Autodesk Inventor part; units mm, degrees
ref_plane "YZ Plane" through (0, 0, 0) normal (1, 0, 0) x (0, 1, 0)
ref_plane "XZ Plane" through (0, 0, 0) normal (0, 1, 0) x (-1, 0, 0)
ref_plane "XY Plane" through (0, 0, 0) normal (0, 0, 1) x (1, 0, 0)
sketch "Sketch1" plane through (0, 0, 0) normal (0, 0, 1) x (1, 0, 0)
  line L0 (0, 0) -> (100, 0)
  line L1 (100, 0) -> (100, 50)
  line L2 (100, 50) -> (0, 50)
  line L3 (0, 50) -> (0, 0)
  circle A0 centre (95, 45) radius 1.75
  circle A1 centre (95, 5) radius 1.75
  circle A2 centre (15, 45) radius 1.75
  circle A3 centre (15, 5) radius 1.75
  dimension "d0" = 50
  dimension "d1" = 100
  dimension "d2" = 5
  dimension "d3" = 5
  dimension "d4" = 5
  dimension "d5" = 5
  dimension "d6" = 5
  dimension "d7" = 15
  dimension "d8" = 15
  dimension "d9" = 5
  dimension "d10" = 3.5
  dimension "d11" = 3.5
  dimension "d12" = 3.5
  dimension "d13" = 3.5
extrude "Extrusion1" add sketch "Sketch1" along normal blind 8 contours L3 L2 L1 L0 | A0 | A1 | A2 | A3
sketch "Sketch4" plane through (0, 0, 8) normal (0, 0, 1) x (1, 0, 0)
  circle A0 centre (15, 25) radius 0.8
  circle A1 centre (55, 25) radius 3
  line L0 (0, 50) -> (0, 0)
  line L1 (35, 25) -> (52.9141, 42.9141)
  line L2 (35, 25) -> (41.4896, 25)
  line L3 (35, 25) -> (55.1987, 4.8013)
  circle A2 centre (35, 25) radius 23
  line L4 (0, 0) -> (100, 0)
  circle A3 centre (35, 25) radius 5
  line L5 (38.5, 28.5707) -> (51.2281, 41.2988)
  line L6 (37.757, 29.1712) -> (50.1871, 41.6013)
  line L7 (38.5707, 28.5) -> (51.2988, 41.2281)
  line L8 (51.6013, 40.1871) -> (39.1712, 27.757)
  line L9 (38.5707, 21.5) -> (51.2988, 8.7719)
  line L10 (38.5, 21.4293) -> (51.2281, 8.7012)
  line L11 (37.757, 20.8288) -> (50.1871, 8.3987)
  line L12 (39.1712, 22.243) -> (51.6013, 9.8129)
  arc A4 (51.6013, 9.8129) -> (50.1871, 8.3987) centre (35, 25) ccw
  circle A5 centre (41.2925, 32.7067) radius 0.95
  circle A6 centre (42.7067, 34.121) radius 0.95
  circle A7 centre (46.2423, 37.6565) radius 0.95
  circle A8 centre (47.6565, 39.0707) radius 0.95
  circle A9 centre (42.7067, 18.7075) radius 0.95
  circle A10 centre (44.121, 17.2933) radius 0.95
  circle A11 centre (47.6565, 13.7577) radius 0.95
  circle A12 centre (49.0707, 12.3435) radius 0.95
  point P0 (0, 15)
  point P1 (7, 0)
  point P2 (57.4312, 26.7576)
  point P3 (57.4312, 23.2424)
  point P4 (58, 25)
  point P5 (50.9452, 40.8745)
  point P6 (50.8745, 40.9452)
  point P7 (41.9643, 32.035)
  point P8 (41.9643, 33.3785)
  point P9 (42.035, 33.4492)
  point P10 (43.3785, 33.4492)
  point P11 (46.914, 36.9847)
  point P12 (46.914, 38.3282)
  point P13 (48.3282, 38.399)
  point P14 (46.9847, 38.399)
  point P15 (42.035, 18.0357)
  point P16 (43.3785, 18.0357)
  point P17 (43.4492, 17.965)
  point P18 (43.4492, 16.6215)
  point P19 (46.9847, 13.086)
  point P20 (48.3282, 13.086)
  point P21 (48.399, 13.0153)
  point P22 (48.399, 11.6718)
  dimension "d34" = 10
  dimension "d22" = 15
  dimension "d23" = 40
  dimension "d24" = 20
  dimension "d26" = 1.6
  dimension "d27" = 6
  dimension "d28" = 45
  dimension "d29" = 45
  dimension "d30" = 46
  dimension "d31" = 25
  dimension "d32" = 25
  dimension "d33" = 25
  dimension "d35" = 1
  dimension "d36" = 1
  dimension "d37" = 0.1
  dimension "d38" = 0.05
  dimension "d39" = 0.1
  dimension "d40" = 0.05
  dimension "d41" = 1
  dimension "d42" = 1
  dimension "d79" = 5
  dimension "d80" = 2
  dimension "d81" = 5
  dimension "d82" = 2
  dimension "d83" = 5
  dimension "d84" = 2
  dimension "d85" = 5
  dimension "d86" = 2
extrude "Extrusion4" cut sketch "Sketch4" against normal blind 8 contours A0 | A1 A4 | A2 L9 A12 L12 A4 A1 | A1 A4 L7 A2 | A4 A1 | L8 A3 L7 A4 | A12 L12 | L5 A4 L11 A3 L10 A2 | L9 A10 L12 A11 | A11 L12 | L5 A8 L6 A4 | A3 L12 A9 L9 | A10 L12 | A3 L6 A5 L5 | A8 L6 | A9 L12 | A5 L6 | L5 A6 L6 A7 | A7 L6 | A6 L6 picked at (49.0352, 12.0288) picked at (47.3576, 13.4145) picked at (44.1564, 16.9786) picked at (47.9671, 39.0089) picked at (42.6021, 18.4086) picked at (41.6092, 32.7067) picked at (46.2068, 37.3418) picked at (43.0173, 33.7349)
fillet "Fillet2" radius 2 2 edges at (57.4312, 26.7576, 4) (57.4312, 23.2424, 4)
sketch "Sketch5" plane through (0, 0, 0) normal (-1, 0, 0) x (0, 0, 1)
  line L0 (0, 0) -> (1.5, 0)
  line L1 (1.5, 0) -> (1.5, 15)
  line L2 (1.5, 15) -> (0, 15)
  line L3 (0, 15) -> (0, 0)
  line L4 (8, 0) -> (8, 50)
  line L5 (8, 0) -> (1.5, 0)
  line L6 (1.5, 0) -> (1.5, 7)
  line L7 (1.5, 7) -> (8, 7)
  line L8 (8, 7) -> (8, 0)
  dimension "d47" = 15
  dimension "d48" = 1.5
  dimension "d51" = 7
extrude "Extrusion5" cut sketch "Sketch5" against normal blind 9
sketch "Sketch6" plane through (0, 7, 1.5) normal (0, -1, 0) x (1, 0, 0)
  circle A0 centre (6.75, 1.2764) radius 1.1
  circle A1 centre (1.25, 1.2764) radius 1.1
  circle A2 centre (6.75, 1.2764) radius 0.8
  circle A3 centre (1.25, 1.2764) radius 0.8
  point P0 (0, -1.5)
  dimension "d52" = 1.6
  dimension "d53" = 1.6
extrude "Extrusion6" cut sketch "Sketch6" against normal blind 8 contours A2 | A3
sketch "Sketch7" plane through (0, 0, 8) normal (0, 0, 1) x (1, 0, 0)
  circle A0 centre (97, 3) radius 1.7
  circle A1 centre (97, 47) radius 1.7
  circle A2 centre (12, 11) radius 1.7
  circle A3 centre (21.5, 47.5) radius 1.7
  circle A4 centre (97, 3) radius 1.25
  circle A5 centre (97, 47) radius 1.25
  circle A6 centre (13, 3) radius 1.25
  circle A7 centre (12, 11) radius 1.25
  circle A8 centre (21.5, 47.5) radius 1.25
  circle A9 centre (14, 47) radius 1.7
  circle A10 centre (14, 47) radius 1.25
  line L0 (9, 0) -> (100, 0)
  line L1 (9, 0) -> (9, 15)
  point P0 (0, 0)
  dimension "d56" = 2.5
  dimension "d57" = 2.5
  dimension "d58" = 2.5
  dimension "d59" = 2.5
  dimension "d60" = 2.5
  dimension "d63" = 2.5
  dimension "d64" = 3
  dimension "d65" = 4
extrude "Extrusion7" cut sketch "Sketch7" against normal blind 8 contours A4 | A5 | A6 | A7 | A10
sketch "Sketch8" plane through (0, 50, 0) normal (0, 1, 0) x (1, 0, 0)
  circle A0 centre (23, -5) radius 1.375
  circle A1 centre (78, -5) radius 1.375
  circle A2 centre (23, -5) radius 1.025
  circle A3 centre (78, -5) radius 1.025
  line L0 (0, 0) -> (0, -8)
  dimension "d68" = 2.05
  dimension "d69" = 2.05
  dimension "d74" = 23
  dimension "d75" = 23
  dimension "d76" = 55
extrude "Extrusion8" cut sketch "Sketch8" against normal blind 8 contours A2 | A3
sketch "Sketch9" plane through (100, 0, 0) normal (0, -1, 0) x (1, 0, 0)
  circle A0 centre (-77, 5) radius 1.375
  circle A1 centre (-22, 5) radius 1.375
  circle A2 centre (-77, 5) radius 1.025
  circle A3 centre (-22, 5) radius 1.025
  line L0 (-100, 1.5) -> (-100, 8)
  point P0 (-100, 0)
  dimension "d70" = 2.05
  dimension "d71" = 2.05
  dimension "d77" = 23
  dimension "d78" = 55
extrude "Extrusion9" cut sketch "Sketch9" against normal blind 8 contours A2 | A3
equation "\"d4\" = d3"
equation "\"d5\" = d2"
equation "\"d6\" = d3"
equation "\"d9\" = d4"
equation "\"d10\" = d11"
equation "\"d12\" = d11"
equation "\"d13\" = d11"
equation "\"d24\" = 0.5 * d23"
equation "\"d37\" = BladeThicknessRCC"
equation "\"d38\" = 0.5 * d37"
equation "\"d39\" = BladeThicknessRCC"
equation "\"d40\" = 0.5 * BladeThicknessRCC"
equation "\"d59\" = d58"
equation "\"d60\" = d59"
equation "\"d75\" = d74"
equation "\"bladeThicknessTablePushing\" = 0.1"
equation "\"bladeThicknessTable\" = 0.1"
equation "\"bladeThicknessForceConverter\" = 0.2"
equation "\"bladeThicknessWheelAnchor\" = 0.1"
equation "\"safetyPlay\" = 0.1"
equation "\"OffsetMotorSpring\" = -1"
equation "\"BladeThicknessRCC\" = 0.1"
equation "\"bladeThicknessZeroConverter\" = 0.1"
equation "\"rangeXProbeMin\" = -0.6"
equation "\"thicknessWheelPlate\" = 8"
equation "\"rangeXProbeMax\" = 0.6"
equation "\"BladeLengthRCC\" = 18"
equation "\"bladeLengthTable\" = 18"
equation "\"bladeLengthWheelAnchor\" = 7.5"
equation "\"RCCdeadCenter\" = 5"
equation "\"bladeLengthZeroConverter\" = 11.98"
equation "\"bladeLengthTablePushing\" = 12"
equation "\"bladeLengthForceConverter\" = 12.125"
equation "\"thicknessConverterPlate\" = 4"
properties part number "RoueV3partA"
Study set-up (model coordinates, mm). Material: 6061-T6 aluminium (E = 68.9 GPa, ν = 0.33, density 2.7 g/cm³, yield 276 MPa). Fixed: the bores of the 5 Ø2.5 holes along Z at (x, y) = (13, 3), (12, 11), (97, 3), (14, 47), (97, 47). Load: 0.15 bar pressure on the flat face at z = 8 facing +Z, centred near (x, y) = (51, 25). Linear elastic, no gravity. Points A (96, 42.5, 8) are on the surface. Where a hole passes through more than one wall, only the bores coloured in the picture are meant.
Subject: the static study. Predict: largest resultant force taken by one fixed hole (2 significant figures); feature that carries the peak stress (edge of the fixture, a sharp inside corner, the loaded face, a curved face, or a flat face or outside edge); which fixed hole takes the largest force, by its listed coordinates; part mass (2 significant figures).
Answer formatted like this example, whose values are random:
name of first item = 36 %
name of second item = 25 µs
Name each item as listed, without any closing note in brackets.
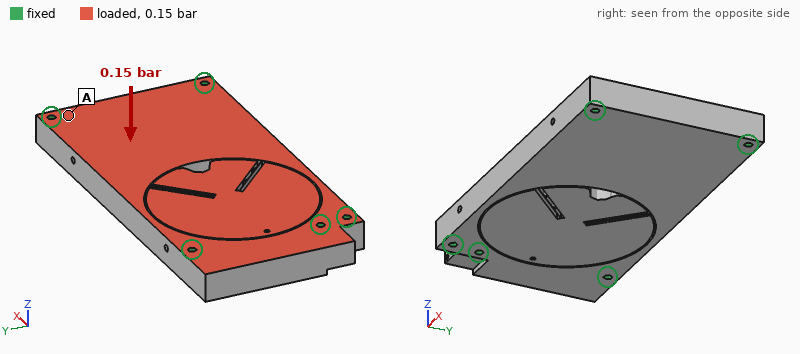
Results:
largest resultant force taken by one fixed hole = 19 N
feature that carries the peak stress = a flat face or outside edge
which fixed hole takes the largest force, by its listed coordinates = (14, 47)
part mass = 100 g
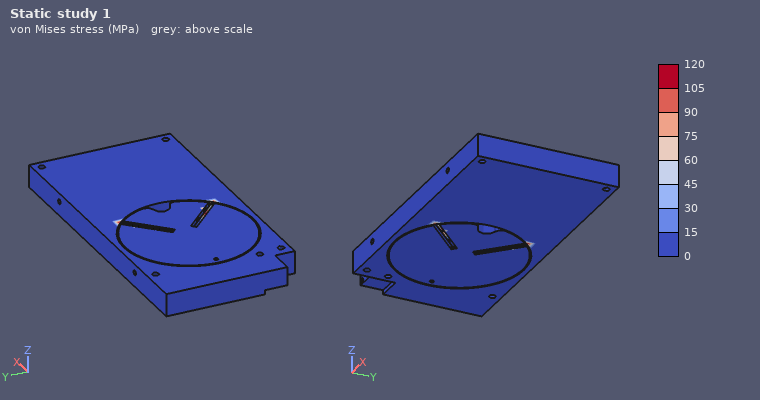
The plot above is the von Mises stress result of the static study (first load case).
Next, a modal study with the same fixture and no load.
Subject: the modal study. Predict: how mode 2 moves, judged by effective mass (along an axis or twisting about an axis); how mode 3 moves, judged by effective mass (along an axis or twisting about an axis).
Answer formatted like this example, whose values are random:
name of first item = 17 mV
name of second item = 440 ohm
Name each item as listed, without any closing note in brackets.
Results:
how mode 2 moves, judged by effective mass = along Z
how mode 3 moves, judged by effective mass = along Y
